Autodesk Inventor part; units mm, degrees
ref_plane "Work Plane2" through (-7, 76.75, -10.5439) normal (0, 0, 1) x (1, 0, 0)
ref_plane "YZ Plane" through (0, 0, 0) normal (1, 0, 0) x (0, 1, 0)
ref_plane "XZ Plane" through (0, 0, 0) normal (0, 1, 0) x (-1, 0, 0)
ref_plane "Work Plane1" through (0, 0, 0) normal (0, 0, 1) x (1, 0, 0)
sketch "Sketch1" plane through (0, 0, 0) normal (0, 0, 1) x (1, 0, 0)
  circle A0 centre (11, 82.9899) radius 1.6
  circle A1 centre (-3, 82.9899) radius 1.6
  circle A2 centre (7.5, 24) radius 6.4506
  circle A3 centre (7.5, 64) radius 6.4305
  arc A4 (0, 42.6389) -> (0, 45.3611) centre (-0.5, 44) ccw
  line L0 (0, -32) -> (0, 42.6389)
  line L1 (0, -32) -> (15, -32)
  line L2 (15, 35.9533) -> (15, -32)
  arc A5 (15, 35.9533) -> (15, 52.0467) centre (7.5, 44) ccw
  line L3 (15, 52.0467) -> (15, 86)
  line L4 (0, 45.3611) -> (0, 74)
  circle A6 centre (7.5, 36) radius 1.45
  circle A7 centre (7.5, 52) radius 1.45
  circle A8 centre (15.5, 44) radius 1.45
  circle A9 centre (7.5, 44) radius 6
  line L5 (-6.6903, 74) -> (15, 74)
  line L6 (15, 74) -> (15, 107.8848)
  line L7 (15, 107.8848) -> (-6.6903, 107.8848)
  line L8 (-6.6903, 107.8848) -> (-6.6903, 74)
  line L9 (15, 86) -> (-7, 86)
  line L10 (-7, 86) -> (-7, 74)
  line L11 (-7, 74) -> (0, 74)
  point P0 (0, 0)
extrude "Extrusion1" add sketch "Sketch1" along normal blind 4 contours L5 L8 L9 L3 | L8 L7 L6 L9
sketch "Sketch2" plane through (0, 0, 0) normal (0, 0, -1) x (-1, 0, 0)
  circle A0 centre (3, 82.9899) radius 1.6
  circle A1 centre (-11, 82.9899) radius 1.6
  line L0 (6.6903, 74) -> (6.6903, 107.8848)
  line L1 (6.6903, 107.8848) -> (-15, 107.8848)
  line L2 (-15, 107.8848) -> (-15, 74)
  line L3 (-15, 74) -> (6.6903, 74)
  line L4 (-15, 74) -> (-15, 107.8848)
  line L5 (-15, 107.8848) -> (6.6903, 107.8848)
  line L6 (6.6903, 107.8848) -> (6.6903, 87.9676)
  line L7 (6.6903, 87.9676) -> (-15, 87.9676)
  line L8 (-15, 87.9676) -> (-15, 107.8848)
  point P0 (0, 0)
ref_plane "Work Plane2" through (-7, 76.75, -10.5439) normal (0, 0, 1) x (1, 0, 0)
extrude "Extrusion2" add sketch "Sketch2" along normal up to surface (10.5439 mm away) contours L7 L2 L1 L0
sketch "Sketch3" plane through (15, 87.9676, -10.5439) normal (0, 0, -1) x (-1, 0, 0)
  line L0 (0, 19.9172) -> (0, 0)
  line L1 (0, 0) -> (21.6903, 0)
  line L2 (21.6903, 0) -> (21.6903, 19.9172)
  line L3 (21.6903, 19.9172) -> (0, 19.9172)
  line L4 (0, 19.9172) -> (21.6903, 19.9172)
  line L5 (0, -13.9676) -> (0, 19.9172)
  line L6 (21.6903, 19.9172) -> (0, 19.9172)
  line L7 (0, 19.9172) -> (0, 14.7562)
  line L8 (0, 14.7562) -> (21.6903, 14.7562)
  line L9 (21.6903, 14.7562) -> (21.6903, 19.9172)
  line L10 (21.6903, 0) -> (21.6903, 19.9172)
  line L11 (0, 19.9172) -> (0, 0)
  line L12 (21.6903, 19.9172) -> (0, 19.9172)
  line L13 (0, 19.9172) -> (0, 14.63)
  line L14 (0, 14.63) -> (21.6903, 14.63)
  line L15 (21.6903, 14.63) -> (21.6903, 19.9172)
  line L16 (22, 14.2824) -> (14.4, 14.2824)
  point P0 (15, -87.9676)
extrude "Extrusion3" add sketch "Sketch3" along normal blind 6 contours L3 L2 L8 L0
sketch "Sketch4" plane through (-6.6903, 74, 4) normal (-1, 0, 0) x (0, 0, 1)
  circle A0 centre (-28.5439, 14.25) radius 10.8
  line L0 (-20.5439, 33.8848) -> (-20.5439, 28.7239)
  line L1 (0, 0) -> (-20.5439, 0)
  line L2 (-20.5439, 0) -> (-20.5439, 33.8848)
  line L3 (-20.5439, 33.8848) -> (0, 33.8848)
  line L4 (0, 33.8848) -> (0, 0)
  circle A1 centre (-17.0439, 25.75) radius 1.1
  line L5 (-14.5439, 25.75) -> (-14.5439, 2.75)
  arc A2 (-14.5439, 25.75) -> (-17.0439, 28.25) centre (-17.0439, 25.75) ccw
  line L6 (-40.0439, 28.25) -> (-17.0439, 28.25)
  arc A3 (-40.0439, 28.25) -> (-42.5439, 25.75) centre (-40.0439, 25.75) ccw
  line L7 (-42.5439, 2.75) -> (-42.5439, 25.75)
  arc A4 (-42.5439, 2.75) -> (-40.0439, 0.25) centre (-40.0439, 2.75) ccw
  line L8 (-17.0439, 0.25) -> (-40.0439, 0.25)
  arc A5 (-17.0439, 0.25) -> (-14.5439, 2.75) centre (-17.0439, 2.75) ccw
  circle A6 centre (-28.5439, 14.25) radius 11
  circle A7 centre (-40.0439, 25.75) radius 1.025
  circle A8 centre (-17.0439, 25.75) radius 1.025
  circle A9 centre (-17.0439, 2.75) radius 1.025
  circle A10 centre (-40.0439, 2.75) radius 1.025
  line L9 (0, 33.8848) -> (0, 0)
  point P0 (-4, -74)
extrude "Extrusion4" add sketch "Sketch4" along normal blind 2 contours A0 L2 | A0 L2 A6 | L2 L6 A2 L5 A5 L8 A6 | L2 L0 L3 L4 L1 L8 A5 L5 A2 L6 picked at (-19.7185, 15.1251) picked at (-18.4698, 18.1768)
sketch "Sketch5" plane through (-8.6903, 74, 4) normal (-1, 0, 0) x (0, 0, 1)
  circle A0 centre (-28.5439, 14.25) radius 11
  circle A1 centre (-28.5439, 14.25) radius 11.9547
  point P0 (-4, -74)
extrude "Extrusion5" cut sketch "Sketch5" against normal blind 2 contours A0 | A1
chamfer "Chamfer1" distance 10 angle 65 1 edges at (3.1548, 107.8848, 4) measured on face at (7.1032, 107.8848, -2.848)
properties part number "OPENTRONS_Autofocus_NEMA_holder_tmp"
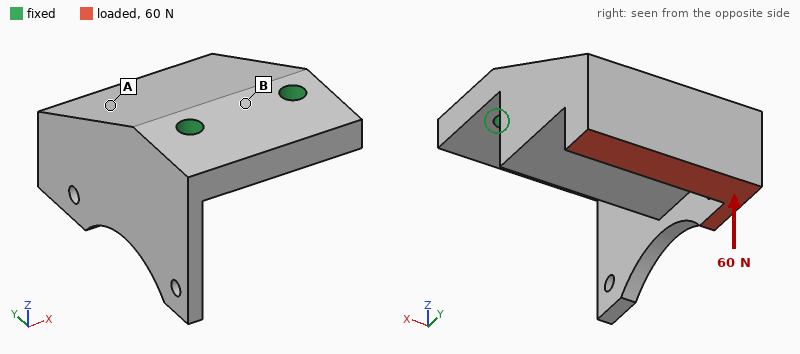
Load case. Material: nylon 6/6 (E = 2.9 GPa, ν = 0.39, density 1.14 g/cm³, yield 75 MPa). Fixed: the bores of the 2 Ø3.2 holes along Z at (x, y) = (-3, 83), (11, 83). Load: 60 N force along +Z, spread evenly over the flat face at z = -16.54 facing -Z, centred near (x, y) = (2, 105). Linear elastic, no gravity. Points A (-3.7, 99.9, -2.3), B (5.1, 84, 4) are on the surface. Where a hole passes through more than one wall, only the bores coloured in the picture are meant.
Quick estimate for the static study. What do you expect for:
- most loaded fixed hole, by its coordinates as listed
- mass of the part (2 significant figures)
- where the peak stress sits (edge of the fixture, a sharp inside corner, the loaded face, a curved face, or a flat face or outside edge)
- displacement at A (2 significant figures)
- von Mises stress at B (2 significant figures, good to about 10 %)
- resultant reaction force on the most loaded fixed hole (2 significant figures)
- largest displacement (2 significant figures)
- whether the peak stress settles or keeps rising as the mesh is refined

(-3, 83)
7.8 g
edge of the fixture
0.22 mm
5.1 MPa
39 N
0.44 mm
keeps rising
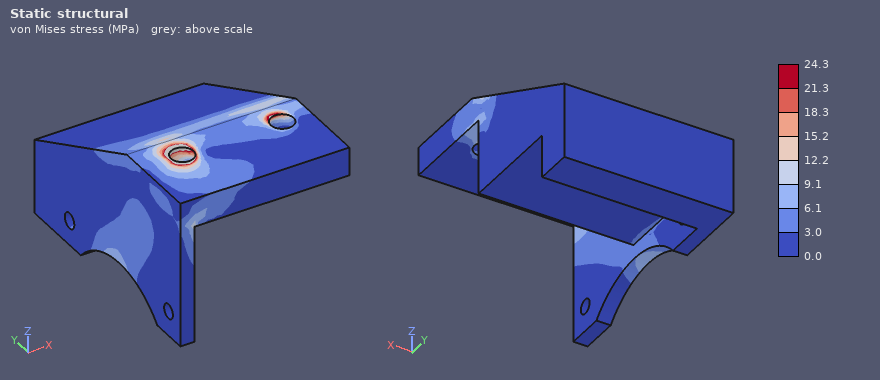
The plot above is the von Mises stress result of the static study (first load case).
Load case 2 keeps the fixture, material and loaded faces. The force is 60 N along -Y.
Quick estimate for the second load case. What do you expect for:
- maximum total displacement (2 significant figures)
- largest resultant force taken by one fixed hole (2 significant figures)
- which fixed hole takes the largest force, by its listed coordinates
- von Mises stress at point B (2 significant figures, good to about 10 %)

0.43 mm
34 N
(-3, 83)
4.3 MPa
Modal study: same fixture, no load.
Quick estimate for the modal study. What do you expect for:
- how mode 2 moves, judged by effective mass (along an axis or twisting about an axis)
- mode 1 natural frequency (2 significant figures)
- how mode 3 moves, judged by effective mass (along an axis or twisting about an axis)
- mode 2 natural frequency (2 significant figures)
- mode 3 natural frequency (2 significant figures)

along X
1100 Hz
along X
2900 Hz
3300 Hz
